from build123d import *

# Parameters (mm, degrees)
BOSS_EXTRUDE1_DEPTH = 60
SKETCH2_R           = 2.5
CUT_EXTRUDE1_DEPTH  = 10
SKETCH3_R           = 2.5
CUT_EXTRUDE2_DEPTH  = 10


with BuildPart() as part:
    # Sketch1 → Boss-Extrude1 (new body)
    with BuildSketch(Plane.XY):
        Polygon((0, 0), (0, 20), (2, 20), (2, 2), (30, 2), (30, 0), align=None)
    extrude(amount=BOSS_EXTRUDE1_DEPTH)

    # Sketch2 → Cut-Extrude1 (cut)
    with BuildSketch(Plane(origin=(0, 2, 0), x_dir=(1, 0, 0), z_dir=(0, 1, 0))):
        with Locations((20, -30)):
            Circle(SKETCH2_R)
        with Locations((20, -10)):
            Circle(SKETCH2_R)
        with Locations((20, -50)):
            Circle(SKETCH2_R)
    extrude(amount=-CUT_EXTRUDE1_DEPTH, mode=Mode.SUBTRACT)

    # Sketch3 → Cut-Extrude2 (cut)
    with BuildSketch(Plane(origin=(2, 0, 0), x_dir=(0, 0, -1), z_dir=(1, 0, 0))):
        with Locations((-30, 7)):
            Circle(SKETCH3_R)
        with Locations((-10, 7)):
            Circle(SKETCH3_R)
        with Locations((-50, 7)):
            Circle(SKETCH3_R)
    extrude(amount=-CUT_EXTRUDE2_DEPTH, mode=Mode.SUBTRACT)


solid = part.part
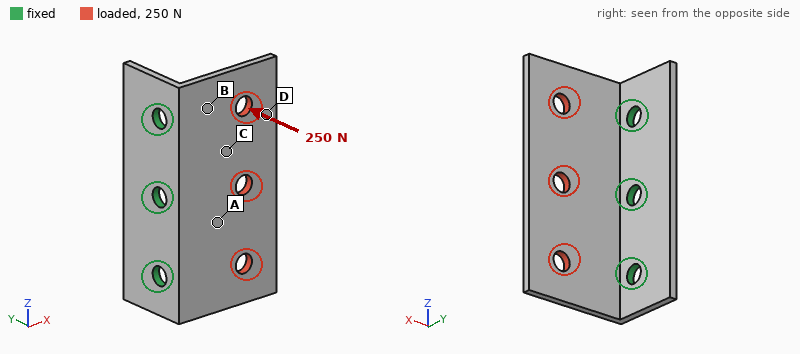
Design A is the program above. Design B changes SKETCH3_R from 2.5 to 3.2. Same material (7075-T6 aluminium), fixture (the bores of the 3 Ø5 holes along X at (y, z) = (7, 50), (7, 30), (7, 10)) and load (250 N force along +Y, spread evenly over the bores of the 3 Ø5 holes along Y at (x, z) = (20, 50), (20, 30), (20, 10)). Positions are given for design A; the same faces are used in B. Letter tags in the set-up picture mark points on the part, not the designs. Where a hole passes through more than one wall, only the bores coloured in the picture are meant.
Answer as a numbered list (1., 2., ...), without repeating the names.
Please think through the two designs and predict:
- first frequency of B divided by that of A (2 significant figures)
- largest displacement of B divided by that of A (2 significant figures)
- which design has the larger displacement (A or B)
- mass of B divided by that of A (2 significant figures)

1. 1.0
2. 0.92
3. A
4. 0.99
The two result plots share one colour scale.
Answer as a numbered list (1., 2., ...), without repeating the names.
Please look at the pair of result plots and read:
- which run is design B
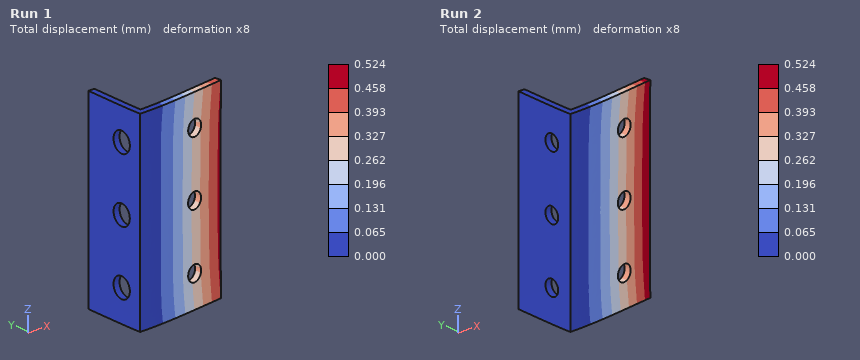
1. Run 1
